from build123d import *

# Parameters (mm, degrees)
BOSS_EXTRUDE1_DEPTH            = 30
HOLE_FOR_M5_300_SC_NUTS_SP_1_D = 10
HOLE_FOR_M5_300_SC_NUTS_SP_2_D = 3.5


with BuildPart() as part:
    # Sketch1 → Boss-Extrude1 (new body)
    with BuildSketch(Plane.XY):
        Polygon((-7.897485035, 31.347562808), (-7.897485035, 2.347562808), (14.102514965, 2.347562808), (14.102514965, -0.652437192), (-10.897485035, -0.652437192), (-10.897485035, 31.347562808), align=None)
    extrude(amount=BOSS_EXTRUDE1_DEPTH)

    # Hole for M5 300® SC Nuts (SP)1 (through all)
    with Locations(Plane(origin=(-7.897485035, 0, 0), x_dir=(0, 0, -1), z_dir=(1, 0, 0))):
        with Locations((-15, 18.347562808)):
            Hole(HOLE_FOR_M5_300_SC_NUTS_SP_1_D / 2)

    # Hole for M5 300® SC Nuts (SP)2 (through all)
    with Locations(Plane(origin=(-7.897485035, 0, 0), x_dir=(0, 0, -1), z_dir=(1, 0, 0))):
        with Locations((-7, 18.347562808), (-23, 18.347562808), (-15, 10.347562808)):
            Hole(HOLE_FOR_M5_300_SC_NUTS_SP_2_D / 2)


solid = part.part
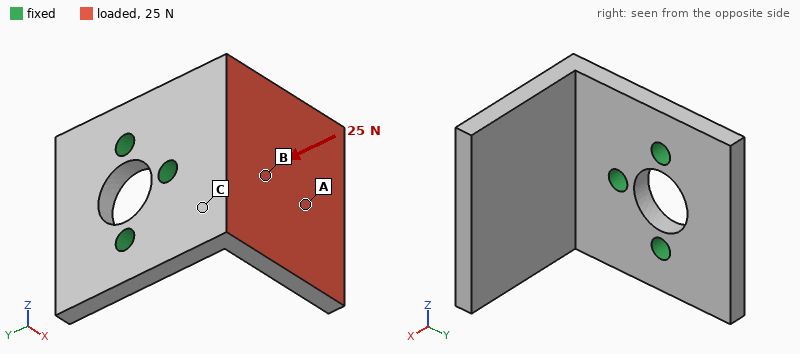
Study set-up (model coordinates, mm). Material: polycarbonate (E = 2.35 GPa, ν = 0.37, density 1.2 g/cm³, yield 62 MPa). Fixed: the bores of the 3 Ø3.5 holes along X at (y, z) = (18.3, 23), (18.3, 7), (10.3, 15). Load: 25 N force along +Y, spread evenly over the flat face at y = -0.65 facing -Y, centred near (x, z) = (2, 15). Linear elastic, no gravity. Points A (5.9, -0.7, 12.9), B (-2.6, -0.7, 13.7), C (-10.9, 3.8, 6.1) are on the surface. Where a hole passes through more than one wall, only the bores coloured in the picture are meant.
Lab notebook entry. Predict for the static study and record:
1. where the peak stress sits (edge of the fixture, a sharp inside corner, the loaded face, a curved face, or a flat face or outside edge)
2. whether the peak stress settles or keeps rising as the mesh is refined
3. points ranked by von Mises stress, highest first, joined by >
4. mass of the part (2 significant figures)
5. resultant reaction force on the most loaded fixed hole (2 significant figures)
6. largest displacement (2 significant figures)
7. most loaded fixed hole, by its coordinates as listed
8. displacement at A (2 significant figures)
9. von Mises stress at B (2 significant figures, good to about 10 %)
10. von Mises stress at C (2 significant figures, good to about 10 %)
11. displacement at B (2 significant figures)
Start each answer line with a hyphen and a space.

- edge of the fixture
- keeps rising
- C > B > A
- 5.4 g
- 21 N
- 0.57 mm
- (10.3, 15)
- 0.36 mm
- 2.8 MPa
- 5.0 MPa
- 0.18 mm
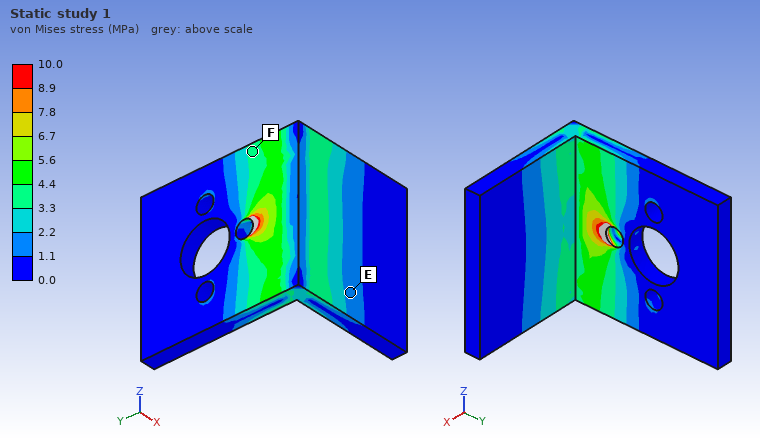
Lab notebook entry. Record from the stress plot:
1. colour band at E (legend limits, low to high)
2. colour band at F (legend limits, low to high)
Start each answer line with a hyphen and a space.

- 1.1 to 2.2 MPa
- 3.3 to 4.4 MPa
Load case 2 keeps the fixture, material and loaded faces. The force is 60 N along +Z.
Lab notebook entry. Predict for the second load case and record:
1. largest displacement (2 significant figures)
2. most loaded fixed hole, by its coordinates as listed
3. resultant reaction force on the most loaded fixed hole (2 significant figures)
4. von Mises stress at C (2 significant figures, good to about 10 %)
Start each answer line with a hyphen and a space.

- 0.54 mm
- (10.3, 15)
- 64 N
- 3.9 MPa
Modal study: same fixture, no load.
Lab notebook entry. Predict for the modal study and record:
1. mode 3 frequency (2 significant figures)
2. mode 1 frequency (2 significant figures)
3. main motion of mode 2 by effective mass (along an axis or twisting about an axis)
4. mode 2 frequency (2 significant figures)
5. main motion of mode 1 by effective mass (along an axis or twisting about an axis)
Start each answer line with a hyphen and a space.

- 2200 Hz
- 770 Hz
- along Z
- 1100 Hz
- along Y
